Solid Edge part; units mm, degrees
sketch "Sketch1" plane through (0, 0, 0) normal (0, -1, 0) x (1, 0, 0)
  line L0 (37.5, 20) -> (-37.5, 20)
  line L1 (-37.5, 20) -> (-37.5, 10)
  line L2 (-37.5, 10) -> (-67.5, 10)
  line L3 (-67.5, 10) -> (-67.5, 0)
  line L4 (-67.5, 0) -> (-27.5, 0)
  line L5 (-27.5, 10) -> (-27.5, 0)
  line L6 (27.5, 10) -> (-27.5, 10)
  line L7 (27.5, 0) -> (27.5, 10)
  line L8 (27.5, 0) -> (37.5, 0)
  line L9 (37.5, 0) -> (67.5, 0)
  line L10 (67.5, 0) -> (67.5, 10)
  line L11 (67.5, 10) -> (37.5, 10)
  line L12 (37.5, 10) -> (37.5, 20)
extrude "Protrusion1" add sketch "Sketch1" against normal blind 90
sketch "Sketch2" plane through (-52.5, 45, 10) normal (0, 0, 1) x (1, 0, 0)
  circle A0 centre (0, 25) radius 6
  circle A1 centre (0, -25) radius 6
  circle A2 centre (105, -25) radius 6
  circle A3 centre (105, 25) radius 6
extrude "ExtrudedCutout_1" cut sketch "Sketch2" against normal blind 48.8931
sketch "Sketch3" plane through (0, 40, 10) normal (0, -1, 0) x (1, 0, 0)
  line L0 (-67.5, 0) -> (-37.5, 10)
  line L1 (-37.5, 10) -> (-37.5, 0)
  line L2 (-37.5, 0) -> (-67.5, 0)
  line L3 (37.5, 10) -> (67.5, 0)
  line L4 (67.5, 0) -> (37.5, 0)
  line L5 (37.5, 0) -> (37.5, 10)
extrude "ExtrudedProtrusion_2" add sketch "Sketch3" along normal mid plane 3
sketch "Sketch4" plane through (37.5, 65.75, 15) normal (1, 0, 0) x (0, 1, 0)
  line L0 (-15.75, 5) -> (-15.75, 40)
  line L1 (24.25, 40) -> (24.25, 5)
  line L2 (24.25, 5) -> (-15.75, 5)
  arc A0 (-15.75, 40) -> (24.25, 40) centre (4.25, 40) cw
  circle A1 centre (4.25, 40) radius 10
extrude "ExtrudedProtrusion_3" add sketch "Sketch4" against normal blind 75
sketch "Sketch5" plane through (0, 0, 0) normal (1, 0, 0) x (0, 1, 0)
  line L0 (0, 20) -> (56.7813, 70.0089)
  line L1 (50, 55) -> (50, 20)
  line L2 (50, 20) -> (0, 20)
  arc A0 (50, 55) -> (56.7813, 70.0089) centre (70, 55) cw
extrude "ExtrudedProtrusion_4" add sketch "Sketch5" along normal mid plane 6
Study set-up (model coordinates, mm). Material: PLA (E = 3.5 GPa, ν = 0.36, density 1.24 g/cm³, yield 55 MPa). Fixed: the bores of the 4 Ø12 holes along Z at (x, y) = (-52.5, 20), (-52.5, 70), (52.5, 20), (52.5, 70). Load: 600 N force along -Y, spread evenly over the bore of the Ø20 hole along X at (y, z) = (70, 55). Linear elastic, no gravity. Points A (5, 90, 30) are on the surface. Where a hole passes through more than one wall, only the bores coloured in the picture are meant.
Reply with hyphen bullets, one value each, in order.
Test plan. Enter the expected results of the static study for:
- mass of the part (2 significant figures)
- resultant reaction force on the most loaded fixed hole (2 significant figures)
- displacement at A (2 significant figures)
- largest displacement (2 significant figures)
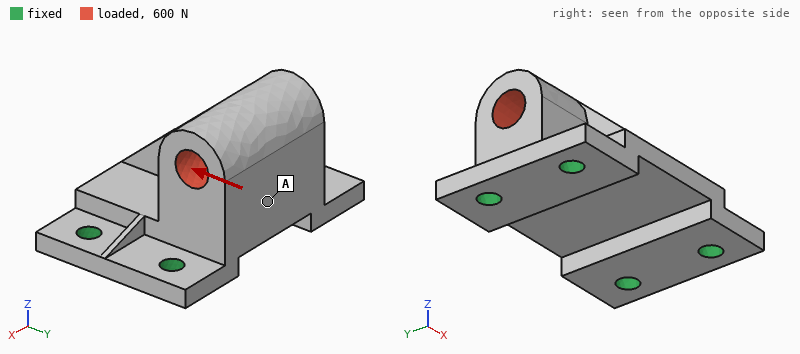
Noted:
- 340 g
- 490 N
- 0.087 mm
- 0.16 mm
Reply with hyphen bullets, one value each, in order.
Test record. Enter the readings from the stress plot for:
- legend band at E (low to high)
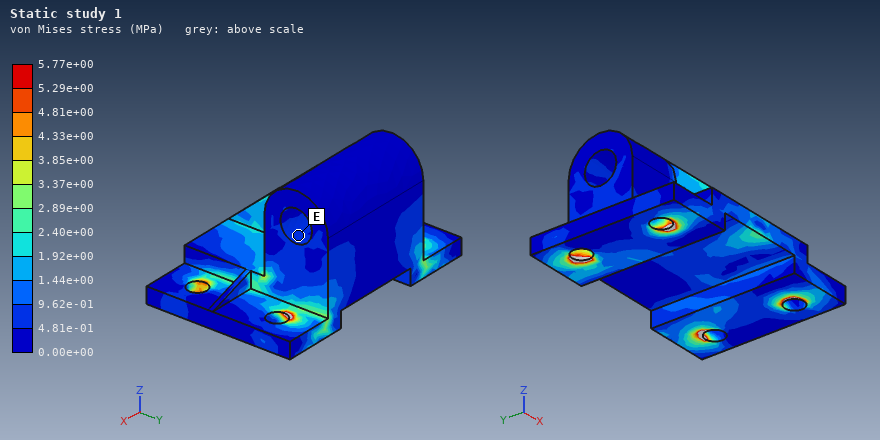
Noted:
- 4.81e-01 to 9.62e-01 MPa
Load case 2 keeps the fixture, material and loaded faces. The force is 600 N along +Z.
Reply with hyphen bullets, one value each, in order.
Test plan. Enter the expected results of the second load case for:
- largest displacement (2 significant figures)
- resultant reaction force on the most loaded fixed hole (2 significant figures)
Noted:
- 47 µm
- 350 N
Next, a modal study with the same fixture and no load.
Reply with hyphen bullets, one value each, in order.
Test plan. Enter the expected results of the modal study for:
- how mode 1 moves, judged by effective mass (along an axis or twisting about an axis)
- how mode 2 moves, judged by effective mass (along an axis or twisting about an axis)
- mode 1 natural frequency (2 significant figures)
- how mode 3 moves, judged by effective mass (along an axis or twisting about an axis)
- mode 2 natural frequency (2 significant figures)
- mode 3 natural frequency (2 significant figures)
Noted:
- along Y
- along X
- 960 Hz
- along Z
- 1700 Hz
- 1700 Hz
